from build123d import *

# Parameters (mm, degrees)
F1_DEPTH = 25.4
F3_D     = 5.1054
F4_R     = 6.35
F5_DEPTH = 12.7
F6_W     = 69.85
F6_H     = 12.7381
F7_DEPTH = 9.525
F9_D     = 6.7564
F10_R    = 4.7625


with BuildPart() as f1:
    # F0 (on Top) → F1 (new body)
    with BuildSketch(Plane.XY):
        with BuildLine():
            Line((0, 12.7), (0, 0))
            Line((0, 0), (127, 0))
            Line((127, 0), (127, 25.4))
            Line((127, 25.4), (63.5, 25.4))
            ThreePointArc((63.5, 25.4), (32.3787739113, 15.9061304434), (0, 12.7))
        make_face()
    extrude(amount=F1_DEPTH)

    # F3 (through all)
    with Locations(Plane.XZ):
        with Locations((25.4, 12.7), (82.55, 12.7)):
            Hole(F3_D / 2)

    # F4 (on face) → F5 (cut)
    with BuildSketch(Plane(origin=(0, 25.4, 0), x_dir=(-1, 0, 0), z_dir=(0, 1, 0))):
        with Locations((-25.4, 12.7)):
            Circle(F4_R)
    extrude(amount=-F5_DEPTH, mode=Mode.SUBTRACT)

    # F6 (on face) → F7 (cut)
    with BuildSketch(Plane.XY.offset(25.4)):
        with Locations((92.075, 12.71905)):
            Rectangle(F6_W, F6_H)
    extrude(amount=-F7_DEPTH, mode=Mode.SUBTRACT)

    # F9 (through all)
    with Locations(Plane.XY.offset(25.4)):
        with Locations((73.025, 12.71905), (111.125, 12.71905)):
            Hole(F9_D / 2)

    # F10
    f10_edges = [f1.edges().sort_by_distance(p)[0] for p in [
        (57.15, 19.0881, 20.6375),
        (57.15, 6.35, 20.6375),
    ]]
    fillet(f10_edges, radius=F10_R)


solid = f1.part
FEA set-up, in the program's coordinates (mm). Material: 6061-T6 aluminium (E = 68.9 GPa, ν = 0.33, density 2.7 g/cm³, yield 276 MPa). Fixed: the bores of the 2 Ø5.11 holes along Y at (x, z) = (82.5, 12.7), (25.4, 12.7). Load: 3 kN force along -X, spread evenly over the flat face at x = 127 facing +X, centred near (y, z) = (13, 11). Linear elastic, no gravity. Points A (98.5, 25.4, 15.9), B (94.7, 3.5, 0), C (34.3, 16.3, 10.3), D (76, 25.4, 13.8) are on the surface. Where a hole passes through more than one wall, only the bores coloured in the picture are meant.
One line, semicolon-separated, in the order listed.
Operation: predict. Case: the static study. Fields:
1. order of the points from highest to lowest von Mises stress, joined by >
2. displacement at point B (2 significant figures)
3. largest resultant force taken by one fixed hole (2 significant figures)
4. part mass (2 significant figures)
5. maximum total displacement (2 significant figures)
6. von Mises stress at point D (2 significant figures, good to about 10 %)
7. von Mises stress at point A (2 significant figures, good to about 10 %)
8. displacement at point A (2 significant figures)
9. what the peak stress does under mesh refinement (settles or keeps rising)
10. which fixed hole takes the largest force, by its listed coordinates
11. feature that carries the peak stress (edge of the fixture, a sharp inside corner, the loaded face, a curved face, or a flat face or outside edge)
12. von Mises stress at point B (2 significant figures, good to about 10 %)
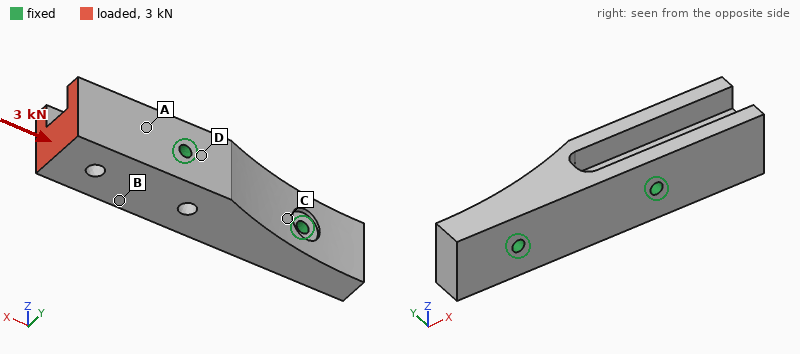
A > B > D > C; 2.2 µm; 2.8 kN; 160 g; 5.8 µm; 2.9 MPa; 6.7 MPa; 1.7 µm; keeps rising; (82.5, 12.7); edge of the fixture; 5.0 MPa
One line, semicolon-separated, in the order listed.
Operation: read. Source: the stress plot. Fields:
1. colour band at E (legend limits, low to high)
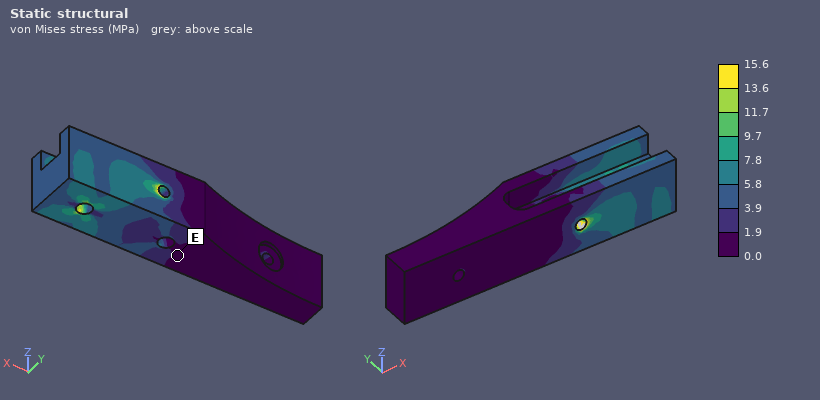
0.0 to 1.9 MPa
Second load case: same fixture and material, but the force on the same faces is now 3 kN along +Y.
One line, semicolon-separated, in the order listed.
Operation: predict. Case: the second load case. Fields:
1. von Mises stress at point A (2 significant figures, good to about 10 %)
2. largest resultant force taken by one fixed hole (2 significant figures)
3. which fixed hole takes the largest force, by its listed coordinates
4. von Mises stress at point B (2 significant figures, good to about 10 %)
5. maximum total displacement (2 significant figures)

39 MPa; 3.4 kN; (82.5, 12.7); 28 MPa; 94 µm
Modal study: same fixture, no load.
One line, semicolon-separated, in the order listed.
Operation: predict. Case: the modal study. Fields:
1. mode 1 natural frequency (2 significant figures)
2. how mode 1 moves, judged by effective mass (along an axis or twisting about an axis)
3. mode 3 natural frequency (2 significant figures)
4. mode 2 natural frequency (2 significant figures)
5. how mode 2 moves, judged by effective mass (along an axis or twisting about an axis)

5900 Hz; along Z; 12 kHz; 7600 Hz; along Y
